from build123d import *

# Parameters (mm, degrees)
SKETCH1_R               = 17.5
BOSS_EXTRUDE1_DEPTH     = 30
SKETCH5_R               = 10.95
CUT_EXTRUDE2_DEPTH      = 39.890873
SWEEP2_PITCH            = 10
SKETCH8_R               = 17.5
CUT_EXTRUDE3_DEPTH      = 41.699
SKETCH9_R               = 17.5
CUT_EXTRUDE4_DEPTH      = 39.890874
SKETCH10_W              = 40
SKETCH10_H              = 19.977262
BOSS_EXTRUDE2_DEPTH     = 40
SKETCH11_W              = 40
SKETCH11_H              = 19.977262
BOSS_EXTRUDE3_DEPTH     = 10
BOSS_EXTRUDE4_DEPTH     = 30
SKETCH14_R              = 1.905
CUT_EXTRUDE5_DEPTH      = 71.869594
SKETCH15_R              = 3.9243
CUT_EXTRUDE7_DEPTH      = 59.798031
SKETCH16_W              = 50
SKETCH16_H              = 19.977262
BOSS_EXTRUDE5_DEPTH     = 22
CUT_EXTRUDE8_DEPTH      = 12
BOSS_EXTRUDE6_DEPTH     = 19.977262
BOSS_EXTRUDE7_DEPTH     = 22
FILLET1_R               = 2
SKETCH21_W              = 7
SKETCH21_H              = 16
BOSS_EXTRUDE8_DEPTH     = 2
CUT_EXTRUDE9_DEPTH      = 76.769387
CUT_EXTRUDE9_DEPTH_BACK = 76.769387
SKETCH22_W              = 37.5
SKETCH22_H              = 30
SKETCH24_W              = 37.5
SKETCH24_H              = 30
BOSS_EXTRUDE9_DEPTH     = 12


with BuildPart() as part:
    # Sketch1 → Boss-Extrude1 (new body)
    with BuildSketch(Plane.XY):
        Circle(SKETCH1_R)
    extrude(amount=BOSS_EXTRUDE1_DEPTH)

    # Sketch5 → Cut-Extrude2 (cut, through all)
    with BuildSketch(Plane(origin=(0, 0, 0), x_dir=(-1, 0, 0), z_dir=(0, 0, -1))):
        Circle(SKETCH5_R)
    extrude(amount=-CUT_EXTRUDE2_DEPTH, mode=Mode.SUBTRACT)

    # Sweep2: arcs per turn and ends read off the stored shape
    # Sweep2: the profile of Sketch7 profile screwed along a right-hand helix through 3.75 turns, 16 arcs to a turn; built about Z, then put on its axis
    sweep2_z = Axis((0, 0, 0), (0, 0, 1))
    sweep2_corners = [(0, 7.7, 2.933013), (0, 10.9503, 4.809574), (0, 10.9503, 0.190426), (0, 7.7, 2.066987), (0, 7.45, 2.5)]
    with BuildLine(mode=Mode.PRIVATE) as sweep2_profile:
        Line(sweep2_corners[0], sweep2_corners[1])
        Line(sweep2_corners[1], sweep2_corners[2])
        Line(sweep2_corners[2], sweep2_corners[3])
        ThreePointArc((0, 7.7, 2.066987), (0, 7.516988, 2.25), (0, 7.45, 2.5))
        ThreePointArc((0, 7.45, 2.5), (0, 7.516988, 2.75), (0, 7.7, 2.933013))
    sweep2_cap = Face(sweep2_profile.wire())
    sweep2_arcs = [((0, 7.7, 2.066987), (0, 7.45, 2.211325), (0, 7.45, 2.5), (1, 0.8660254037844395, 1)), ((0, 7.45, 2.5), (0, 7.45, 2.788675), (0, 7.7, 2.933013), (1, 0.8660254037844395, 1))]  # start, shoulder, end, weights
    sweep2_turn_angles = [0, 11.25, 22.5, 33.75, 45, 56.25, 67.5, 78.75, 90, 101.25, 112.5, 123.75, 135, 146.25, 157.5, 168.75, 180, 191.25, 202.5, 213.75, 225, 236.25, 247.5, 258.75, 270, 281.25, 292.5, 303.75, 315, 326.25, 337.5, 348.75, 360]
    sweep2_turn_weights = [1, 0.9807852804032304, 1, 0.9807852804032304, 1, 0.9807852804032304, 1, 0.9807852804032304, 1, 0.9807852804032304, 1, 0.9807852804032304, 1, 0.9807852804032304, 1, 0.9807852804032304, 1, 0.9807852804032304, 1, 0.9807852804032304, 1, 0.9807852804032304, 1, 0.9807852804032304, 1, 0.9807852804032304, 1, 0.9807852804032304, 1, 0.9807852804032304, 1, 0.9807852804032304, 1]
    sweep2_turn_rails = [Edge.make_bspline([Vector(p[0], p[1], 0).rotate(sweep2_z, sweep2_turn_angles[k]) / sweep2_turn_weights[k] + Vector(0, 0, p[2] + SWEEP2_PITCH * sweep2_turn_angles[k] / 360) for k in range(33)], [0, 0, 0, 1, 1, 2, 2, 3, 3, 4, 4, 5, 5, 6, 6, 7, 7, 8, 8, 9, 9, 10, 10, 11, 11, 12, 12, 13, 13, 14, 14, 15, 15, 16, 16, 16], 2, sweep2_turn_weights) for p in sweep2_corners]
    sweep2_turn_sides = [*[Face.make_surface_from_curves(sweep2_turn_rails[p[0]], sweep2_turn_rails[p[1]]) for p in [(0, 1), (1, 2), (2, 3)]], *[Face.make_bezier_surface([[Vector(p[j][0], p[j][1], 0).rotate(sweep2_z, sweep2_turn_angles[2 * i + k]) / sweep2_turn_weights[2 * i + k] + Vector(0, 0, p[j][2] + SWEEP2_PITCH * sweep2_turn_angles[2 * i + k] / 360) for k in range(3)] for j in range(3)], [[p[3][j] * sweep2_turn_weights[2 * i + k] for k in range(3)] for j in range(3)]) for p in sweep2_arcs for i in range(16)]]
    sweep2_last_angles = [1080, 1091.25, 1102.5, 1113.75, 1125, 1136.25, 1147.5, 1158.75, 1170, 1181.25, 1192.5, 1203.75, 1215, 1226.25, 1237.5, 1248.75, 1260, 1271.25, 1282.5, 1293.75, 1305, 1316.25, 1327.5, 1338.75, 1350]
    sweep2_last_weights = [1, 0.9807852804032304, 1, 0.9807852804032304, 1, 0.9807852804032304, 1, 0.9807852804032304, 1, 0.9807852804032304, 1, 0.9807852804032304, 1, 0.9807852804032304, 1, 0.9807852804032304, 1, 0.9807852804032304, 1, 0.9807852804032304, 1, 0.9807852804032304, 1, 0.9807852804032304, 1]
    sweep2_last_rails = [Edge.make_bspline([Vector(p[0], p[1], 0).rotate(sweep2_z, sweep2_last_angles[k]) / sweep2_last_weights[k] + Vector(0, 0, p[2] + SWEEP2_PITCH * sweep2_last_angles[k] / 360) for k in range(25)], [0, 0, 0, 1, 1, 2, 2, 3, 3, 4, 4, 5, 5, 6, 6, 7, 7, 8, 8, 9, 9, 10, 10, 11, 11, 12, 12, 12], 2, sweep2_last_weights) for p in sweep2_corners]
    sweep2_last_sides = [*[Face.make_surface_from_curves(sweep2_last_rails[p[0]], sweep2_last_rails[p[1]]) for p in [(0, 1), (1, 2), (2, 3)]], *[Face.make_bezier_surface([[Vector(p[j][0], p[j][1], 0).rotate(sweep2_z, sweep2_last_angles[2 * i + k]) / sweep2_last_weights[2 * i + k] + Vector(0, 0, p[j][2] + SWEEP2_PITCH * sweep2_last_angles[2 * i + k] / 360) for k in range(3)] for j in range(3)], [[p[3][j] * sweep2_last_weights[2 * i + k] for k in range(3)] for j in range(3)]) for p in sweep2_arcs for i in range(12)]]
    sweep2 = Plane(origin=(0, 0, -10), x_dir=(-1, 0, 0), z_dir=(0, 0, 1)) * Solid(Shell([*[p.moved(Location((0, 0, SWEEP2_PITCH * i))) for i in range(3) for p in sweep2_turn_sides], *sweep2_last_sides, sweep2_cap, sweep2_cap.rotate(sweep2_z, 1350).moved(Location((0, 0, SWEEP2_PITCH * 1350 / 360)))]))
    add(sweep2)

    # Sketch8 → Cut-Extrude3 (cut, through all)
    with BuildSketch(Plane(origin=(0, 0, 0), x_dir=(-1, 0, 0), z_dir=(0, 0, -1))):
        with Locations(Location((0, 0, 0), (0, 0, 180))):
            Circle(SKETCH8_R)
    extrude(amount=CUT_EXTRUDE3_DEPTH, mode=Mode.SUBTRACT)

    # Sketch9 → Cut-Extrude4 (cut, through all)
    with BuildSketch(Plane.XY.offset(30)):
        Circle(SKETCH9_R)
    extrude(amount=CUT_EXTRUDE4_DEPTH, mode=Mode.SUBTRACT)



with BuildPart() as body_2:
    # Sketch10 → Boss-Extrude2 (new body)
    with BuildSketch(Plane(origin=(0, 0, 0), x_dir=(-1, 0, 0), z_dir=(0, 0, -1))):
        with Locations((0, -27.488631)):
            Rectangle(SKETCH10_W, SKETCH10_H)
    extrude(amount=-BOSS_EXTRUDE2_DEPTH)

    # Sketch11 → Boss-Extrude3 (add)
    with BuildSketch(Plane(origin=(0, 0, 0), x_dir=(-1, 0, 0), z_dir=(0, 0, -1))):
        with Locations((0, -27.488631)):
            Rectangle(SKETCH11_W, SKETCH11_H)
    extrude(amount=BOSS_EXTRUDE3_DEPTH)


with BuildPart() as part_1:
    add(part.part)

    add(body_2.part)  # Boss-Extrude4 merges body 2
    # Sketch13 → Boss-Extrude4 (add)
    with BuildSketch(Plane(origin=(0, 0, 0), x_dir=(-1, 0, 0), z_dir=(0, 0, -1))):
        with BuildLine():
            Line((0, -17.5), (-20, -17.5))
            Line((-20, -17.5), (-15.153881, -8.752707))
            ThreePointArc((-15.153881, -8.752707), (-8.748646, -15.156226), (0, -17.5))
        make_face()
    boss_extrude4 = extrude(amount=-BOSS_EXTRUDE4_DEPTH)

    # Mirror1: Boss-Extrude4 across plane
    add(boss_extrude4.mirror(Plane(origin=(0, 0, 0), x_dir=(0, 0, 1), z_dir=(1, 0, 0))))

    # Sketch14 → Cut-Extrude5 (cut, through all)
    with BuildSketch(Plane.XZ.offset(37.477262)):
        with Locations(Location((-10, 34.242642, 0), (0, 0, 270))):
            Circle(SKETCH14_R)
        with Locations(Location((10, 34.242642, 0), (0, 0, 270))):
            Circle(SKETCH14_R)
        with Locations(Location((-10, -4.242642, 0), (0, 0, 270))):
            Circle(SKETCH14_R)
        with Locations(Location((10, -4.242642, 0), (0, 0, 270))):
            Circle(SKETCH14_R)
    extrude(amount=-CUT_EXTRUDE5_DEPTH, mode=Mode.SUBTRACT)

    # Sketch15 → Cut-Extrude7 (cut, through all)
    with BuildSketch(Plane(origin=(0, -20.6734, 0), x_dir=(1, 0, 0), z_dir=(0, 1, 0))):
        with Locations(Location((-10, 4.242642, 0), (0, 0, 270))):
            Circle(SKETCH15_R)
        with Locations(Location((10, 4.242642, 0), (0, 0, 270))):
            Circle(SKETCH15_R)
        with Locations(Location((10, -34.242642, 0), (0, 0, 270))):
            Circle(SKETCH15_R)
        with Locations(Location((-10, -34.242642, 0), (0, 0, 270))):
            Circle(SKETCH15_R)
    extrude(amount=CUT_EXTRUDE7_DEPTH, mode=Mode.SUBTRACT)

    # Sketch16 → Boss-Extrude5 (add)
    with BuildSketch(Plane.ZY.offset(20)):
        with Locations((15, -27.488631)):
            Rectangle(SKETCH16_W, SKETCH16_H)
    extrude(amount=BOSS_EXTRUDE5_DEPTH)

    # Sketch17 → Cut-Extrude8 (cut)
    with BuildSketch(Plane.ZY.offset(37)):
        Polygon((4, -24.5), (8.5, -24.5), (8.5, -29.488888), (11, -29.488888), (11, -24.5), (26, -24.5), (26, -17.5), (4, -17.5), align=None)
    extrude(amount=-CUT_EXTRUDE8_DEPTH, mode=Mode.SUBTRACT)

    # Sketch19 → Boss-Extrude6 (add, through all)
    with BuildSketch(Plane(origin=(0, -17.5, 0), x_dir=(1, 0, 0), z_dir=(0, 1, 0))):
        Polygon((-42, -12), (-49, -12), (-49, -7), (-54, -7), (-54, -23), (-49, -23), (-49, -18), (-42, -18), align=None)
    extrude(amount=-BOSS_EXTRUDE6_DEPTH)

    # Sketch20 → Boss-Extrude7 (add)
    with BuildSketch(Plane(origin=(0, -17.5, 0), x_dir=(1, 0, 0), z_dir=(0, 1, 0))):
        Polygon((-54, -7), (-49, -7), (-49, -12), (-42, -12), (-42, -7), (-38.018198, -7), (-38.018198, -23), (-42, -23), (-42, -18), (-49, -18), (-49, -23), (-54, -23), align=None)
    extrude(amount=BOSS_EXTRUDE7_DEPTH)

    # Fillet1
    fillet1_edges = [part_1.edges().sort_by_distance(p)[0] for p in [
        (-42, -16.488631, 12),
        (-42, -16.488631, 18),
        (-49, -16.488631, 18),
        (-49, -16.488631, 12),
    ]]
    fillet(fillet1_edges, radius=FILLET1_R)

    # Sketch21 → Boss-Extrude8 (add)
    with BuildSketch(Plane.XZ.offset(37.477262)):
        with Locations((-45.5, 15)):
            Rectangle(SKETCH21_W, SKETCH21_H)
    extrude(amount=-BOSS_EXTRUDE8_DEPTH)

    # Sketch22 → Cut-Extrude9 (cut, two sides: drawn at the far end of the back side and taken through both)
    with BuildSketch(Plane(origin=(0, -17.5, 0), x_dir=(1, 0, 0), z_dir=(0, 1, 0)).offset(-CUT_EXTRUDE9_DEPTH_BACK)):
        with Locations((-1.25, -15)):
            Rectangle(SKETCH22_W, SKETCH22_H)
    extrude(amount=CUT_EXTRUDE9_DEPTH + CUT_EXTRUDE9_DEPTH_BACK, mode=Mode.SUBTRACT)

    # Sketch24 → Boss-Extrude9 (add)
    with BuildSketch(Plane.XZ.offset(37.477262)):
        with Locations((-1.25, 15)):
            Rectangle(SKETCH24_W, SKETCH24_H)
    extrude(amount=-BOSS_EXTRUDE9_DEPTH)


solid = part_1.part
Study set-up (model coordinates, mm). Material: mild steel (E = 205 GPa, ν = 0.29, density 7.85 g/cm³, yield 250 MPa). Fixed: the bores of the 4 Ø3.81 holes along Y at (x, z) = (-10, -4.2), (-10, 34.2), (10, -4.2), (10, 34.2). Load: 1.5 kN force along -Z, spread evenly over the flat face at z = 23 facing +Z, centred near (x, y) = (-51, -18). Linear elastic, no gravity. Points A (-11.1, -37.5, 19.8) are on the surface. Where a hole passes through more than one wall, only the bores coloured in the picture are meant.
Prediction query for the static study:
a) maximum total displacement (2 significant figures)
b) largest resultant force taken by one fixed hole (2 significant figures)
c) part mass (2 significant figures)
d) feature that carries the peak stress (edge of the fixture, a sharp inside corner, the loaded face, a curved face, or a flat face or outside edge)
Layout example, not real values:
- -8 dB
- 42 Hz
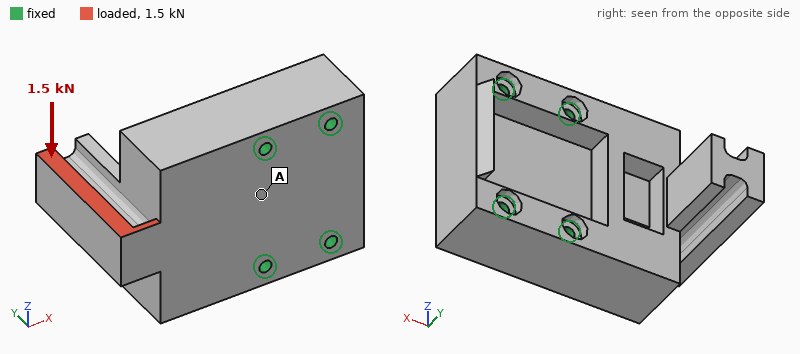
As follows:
- 27 µm
- 1.6 kN
- 440 g
- a curved face
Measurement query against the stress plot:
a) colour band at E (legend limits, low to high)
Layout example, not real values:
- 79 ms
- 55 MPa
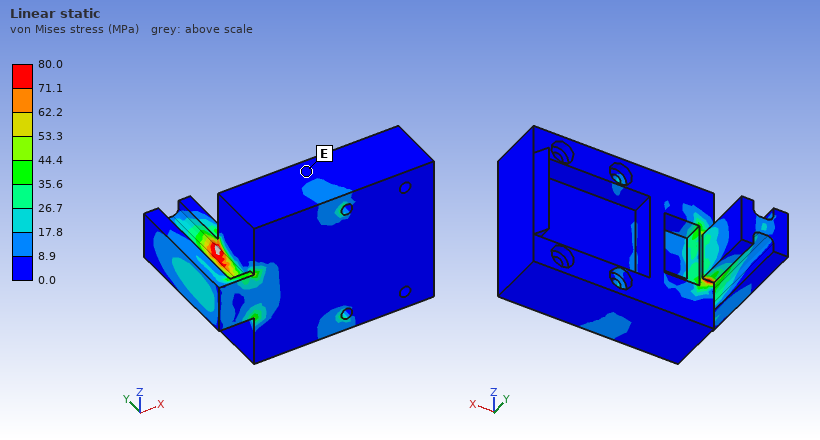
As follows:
- 0.0 to 8.9 MPa
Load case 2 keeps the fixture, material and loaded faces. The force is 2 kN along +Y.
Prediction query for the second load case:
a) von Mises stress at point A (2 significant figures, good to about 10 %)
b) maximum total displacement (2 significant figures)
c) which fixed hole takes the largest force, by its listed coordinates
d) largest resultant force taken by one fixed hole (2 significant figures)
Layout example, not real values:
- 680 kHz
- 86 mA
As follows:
- 21 MPa
- 48 µm
- (-10, 34.2)
- 1.9 kN
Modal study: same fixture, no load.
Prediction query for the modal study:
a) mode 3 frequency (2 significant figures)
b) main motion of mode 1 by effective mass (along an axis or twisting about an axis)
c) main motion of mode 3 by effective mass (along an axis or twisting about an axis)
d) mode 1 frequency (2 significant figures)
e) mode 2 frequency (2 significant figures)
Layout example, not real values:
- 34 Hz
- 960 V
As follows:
- 9400 Hz
- along Y
- along Y
- 4800 Hz
- 7100 Hz
